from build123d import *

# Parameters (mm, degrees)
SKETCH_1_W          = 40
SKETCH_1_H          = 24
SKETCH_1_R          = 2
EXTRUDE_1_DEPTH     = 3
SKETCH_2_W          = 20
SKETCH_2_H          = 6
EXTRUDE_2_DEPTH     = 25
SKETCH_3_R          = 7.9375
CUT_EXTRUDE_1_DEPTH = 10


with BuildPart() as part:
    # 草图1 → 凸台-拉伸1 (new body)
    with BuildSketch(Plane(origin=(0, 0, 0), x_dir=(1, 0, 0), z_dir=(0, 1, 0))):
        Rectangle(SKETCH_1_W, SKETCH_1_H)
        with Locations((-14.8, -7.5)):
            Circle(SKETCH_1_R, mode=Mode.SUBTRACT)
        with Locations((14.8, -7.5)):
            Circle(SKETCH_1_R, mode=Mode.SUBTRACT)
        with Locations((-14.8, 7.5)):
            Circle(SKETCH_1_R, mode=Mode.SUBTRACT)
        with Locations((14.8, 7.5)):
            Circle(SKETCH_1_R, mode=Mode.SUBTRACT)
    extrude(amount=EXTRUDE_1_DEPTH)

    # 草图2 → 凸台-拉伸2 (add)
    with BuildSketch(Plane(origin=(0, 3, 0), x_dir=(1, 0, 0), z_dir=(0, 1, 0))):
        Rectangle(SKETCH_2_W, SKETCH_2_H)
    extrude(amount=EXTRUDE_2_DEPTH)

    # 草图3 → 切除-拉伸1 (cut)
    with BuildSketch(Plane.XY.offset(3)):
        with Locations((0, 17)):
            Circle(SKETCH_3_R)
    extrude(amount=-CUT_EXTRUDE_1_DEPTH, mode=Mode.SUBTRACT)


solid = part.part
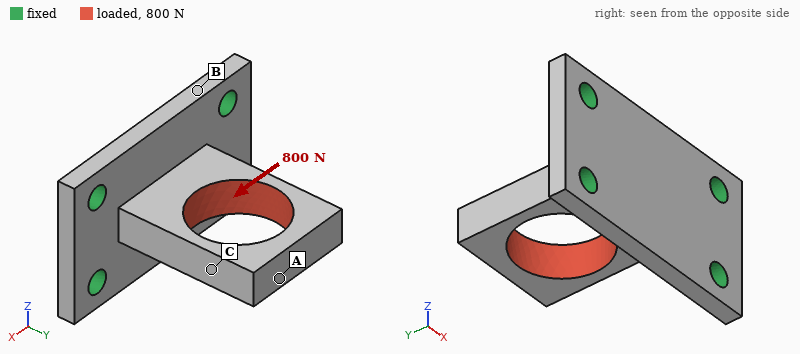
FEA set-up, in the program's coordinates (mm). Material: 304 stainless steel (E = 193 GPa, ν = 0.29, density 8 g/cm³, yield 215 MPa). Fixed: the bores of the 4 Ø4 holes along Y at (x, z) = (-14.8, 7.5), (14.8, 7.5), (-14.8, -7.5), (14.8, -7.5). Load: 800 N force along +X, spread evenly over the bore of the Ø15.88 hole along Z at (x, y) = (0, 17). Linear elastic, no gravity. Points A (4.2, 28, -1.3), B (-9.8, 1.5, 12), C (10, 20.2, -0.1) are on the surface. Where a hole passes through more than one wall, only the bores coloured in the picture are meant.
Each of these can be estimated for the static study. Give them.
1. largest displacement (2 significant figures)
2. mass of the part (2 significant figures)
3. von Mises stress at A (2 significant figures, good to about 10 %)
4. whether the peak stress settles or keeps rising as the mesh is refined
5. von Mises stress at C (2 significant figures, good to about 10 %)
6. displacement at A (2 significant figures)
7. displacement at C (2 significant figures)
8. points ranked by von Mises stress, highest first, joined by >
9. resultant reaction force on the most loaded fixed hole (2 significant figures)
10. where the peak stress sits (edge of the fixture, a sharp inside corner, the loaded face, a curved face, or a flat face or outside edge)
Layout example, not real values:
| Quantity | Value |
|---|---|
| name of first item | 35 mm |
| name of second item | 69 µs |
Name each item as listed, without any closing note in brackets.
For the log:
| Quantity | Value |
|---|---|
| largest displacement | 33 µm |
| mass of the part | 36 g |
| von Mises stress at A | 30 MPa |
| whether the peak stress settles or keeps rising as the mesh is refined | keeps rising |
| von Mises stress at C | 69 MPa |
| displacement at A | 32 µm |
| displacement at C | 26 µm |
| points ranked by von Mises stress, highest first, joined by > | C > A > B |
| resultant reaction force on the most loaded fixed hole | 340 N |
| where the peak stress sits | edge of the fixture |
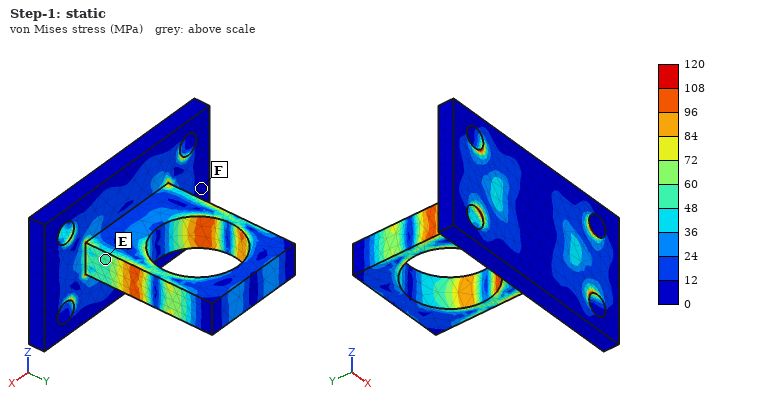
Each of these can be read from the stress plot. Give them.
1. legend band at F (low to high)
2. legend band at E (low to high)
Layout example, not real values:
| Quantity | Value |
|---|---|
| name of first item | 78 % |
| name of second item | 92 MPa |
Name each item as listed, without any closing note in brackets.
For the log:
| Quantity | Value |
|---|---|
| legend band at F | 0 to 12 MPa |
| legend band at E | 48 to 60 MPa |
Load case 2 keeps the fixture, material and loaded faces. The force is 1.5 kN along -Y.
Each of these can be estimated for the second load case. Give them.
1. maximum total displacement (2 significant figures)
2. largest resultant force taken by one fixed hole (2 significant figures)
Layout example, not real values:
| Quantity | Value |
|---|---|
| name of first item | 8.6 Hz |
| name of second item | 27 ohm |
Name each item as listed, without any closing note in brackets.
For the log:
| Quantity | Value |
|---|---|
| maximum total displacement | 13 µm |
| largest resultant force taken by one fixed hole | 390 N |
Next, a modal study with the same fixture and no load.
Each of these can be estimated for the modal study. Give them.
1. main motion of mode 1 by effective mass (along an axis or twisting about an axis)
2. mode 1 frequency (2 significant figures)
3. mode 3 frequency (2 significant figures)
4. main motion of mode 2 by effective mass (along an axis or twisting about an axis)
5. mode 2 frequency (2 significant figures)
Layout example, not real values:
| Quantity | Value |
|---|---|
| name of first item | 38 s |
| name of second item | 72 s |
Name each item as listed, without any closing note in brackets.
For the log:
| Quantity | Value |
|---|---|
| main motion of mode 1 by effective mass | along Z |
| mode 1 frequency | 4900 Hz |
| mode 3 frequency | 11 kHz |
| main motion of mode 2 by effective mass | along X |
| mode 2 frequency | 7900 Hz |
